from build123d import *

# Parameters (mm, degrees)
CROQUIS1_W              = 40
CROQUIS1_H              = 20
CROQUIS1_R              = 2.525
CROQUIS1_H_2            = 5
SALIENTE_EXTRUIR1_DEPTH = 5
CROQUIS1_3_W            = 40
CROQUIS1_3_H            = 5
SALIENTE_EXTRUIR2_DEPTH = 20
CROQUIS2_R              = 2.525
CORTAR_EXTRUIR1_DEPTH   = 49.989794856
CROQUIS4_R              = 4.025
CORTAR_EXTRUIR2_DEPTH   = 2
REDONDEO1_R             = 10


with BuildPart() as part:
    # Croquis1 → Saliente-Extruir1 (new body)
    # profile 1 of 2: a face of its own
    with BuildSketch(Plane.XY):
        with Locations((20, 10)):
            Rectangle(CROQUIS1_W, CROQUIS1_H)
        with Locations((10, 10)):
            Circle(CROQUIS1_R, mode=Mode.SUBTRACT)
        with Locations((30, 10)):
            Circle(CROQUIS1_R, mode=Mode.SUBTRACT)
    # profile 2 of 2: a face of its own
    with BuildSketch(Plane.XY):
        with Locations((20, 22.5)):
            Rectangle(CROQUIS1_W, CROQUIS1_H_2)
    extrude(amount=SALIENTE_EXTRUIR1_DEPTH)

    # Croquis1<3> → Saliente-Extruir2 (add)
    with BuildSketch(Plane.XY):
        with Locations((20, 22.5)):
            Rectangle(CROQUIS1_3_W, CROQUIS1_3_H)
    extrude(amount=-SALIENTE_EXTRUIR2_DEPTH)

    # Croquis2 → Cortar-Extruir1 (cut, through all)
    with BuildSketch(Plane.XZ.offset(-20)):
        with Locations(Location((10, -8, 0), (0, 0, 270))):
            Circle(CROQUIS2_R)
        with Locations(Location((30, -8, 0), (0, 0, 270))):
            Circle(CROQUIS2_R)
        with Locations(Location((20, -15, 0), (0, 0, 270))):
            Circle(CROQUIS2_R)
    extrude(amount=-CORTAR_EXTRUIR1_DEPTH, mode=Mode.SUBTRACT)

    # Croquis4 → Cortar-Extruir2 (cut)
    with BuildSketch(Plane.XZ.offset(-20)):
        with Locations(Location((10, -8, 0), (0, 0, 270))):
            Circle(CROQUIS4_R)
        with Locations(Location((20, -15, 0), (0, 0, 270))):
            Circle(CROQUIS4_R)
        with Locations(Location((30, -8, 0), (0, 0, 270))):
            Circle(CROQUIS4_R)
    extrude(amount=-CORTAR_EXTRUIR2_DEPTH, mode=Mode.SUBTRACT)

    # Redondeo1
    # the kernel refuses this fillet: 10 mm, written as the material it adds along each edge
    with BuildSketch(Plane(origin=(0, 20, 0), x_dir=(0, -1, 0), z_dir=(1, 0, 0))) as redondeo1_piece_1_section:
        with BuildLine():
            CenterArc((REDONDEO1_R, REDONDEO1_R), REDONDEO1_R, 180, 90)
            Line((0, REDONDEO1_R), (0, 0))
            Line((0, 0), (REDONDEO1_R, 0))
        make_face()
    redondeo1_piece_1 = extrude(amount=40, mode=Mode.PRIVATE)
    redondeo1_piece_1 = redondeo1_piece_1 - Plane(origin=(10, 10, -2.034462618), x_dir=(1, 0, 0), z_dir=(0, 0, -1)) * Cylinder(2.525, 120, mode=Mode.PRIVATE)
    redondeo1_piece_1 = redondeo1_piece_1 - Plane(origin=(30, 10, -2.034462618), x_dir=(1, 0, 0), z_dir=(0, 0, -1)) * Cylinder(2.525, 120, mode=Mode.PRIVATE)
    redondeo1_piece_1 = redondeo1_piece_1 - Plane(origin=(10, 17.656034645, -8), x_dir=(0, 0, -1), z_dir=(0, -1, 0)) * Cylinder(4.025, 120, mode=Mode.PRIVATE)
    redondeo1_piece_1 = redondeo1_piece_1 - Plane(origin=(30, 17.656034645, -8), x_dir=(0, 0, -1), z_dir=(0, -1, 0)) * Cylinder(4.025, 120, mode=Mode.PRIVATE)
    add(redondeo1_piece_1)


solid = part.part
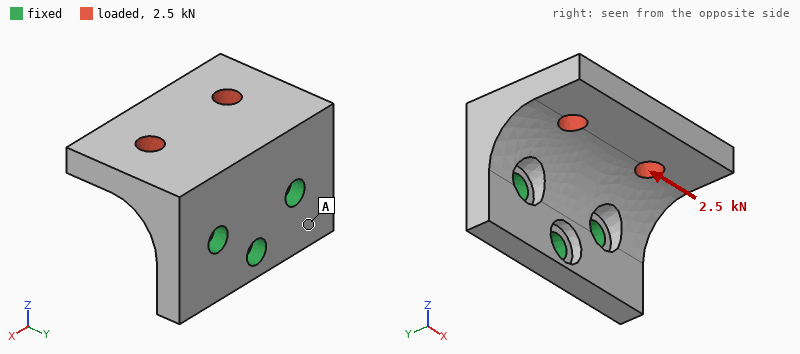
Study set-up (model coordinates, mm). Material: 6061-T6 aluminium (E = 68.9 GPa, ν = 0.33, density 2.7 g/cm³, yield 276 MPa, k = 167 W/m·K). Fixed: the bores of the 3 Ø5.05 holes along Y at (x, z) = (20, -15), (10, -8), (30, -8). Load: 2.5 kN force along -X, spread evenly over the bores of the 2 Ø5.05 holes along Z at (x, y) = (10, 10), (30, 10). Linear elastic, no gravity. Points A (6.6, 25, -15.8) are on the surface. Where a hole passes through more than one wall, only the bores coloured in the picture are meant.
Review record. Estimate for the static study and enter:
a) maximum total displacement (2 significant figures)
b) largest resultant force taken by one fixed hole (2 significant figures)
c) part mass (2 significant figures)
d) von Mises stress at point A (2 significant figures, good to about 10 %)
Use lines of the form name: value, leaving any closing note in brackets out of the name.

maximum total displacement: 52 µm
largest resultant force taken by one fixed hole: 2.2 kN
part mass: 25 g
von Mises stress at point A: 20 MPa
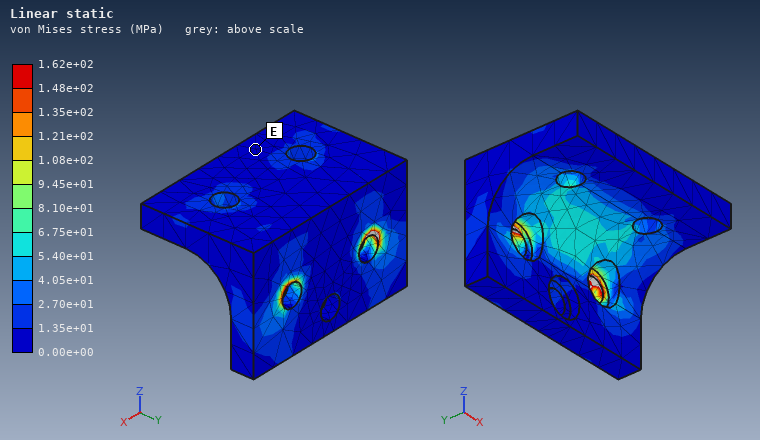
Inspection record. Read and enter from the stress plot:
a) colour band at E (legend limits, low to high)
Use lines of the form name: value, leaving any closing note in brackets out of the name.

colour band at E: 0.00e+00 to 1.35e+01 MPa
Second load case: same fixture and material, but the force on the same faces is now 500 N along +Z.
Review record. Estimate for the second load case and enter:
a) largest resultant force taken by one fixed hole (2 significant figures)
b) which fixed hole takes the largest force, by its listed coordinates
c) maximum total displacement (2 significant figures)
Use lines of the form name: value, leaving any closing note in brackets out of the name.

largest resultant force taken by one fixed hole: 460 N
which fixed hole takes the largest force, by its listed coordinates: (20, -15)
maximum total displacement: 46 µm
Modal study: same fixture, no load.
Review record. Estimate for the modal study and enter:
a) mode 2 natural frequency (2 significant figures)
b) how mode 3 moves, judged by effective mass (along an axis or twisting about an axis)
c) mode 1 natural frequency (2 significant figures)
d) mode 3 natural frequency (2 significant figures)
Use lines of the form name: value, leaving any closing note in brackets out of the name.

mode 2 natural frequency: 9600 Hz
how mode 3 moves, judged by effective mass: along X
mode 1 natural frequency: 5400 Hz
mode 3 natural frequency: 15 kHz
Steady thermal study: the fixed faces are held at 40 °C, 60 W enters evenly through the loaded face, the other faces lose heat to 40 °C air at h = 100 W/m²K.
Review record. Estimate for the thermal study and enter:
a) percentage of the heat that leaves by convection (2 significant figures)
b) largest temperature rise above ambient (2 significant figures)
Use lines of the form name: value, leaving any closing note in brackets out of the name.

percentage of the heat that leaves by convection: 11 %
largest temperature rise above ambient: 34 K
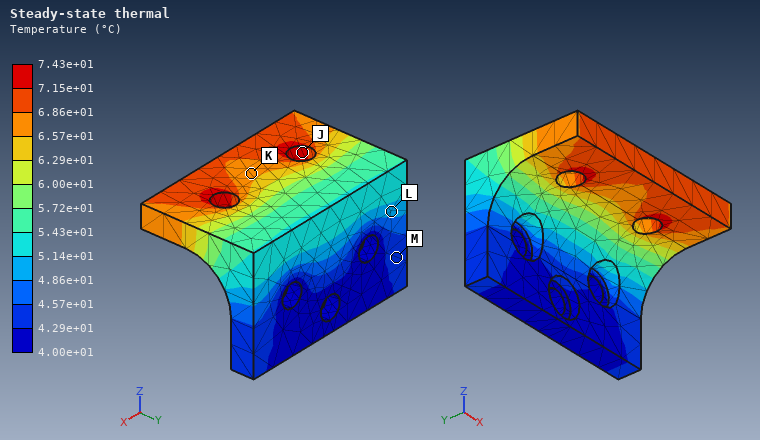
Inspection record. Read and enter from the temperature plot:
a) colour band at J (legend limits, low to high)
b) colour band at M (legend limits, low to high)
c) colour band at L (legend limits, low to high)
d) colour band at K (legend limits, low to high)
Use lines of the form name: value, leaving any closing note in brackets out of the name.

colour band at J: 7.15e+01 to 7.43e+01 °C
colour band at M: 4.29e+01 to 4.57e+01 °C
colour band at L: 4.86e+01 to 5.14e+01 °C
colour band at K: 6.57e+01 to 6.86e+01 °C
